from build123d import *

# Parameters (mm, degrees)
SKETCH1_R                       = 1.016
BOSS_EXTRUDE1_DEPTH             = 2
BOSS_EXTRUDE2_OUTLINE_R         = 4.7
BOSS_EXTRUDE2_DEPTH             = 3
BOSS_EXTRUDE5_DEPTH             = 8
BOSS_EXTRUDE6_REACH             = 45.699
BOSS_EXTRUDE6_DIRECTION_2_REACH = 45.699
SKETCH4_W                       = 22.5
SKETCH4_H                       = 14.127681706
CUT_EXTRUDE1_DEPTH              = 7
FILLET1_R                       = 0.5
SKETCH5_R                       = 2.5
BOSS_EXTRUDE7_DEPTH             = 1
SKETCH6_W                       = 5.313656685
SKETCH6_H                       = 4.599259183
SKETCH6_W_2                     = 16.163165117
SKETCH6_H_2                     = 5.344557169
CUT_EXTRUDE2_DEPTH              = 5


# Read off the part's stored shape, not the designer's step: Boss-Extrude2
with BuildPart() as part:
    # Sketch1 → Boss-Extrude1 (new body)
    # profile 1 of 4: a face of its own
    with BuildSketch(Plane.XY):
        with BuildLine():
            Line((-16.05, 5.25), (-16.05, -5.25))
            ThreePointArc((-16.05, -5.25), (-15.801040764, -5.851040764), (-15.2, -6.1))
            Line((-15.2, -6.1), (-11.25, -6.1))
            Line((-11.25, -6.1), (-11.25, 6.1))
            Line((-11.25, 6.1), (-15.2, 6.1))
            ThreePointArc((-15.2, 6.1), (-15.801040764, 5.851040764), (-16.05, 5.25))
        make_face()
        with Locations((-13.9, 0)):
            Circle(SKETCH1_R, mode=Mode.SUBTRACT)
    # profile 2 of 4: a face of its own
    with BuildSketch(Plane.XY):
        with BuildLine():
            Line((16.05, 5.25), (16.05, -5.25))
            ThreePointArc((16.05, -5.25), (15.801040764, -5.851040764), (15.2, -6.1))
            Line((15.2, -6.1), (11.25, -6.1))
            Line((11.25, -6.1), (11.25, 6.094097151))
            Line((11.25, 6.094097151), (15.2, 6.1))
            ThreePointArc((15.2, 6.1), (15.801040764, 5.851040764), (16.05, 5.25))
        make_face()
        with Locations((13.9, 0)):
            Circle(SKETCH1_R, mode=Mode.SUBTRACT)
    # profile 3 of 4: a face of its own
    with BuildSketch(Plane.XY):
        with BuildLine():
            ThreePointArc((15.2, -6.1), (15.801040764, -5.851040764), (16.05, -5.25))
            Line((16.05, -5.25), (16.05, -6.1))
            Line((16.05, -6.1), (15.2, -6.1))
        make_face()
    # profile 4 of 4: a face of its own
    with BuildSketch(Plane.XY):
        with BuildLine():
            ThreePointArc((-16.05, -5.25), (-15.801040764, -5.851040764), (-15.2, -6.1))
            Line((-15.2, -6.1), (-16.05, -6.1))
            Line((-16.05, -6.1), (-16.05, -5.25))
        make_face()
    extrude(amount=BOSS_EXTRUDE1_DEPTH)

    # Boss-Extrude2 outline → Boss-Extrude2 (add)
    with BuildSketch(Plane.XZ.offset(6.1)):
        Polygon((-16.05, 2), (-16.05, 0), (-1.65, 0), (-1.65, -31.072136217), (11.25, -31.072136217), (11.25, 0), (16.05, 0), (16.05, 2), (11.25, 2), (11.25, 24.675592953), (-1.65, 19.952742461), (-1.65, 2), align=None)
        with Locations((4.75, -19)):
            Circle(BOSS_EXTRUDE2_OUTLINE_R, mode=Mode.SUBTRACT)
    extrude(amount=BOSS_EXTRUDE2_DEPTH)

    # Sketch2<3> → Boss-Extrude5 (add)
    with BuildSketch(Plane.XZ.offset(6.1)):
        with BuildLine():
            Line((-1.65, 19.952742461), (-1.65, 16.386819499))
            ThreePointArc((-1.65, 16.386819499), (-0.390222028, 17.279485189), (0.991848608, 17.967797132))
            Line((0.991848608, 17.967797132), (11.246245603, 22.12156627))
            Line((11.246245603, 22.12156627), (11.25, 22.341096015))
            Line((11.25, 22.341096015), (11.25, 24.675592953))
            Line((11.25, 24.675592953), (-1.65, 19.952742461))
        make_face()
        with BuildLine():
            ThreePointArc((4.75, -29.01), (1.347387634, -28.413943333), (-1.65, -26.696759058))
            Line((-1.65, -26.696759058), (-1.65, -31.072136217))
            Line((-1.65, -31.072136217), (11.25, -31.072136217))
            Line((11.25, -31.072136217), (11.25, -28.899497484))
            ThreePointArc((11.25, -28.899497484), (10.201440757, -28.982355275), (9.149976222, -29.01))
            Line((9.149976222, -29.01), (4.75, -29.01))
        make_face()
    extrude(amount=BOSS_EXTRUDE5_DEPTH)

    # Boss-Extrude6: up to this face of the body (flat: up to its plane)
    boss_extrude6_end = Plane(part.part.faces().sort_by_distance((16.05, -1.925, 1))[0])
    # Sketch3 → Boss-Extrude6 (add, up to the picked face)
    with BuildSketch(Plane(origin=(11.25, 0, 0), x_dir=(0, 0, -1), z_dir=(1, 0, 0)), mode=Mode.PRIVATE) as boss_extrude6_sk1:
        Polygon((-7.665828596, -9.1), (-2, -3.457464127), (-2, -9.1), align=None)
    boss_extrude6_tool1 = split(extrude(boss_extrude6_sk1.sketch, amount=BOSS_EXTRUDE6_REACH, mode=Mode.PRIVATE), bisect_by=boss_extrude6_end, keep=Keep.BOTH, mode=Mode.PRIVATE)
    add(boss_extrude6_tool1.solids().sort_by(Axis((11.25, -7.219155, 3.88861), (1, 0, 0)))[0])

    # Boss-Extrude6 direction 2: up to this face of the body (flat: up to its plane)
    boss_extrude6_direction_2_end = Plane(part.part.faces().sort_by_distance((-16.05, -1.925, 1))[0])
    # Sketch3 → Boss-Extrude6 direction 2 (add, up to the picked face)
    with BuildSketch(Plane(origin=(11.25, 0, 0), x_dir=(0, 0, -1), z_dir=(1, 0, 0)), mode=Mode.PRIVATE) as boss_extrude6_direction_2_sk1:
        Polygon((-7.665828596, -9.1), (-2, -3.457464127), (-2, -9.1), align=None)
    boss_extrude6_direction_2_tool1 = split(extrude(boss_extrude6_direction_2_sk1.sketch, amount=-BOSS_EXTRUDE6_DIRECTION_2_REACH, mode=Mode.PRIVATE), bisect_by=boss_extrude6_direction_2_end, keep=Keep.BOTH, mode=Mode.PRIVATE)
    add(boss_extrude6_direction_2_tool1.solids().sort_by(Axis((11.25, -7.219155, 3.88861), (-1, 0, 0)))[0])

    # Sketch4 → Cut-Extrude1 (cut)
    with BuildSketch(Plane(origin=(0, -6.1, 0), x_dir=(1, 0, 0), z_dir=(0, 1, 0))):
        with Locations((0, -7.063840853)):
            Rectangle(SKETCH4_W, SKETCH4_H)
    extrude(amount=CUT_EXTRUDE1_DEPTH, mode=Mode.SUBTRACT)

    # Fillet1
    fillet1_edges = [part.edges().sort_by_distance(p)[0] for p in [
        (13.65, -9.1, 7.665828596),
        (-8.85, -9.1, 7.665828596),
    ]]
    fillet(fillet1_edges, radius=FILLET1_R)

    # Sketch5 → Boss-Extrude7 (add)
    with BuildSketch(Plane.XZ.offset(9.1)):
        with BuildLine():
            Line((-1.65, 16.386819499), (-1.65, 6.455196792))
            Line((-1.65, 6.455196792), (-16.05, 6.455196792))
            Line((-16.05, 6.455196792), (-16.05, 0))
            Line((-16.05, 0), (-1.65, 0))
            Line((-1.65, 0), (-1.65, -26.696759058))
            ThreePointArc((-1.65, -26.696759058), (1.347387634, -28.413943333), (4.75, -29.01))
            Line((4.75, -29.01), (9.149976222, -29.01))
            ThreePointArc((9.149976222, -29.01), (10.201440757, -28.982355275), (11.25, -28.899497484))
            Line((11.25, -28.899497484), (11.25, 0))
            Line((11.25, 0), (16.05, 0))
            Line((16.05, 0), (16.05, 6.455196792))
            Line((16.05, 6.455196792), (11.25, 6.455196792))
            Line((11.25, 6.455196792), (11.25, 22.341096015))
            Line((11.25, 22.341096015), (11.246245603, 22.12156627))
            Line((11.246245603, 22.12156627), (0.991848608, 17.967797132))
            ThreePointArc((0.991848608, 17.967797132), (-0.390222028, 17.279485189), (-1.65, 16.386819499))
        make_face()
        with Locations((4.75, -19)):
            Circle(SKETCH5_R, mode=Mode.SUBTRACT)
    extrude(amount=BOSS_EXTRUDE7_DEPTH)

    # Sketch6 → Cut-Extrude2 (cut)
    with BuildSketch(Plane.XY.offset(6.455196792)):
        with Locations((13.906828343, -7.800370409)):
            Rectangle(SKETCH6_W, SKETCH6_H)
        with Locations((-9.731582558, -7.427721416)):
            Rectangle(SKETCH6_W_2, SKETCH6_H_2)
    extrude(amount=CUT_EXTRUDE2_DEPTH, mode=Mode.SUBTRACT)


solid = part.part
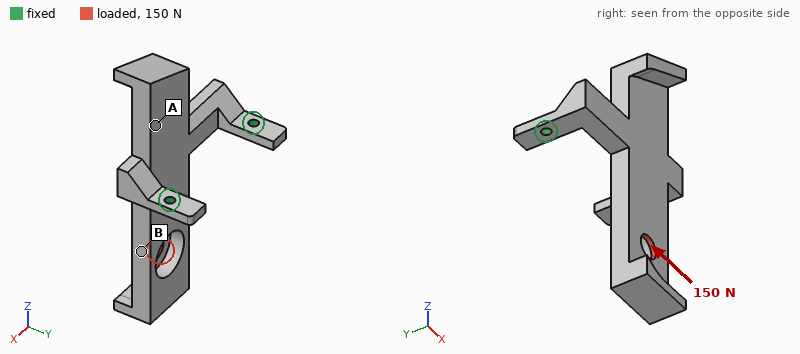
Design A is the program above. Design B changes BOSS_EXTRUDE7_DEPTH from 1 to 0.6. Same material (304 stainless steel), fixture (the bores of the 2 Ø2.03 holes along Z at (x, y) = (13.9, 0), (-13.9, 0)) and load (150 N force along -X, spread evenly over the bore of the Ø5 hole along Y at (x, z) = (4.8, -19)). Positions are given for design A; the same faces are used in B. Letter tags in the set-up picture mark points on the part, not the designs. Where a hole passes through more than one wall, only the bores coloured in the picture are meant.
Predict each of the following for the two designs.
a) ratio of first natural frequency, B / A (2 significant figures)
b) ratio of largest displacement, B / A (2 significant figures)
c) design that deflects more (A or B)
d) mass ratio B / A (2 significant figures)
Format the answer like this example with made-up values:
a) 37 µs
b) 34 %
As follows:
a) 1.0
b) 1.1
c) B
d) 0.92
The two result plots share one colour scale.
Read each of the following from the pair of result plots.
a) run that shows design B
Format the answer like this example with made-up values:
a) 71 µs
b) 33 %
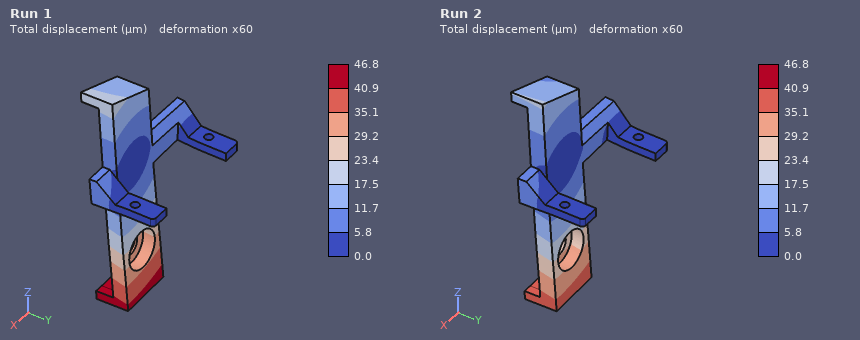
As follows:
a) Run 1
